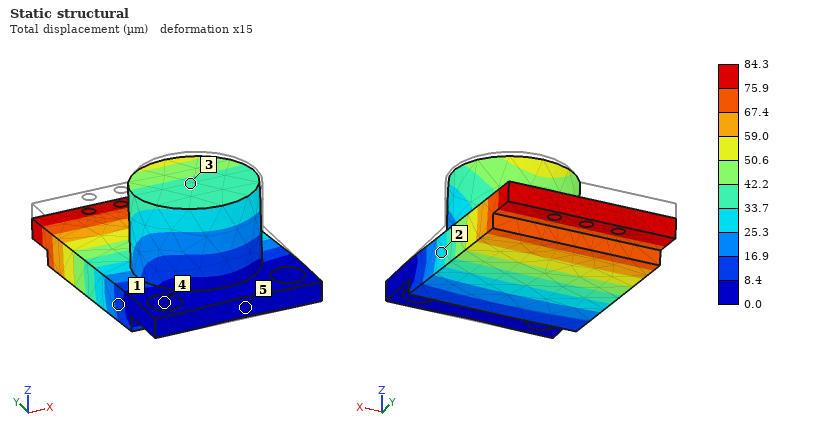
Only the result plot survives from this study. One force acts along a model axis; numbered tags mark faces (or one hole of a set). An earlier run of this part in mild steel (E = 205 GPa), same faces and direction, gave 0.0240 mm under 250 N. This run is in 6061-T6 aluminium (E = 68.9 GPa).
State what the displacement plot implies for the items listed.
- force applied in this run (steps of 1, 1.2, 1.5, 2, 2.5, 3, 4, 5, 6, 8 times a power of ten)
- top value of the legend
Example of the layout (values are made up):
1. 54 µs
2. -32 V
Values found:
1. 300 N
2. 84.3 µm
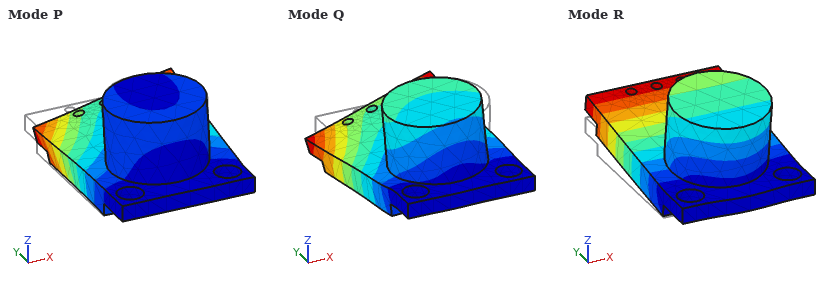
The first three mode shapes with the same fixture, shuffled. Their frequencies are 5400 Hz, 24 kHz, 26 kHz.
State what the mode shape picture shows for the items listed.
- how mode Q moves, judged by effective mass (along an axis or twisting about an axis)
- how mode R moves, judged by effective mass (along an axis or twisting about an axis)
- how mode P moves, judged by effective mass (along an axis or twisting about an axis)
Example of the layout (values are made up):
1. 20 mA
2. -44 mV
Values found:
1. along X
2. along Z
3. along X
